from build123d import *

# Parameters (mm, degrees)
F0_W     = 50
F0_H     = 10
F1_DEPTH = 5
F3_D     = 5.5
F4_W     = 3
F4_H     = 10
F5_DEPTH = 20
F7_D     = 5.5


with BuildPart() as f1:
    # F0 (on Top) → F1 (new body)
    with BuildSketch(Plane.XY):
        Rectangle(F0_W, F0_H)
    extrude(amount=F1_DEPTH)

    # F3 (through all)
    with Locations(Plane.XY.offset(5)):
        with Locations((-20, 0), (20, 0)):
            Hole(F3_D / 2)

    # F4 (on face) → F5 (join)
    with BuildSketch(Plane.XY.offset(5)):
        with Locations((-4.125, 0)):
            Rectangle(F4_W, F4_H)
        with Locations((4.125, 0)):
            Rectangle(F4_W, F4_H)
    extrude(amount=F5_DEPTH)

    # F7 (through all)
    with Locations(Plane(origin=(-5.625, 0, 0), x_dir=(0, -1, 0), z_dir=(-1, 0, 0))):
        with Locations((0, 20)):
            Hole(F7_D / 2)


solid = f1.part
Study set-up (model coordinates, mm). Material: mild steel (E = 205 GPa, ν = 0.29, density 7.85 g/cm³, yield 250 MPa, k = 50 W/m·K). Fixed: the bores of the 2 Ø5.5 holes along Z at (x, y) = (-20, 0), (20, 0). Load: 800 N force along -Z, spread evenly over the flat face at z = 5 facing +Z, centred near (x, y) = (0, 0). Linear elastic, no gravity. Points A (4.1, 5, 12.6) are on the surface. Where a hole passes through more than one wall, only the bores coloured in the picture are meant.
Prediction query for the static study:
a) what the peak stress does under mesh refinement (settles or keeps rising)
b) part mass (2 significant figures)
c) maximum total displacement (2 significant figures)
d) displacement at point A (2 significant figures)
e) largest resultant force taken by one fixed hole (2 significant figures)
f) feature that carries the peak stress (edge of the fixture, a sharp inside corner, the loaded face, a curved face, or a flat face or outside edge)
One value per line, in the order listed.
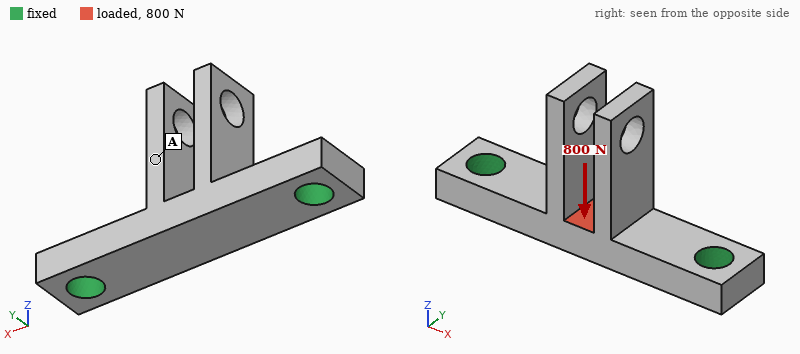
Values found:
keeps rising
26 g
17 µm
11 µm
400 N
edge of the fixture
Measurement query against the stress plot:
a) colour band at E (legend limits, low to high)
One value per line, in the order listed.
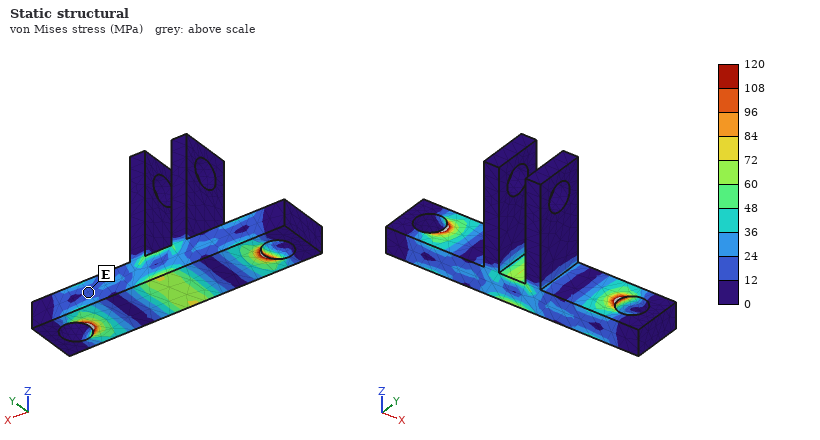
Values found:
12 to 24 MPa
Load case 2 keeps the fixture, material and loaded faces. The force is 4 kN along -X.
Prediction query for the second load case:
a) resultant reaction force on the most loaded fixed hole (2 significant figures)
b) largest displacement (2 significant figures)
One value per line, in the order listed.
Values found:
2.0 kN
9.9 µm
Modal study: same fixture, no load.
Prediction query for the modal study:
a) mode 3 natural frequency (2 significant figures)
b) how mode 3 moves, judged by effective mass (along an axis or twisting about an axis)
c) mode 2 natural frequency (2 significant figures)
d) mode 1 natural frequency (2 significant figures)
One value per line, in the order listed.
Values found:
6800 Hz
along Y
6000 Hz
5800 Hz
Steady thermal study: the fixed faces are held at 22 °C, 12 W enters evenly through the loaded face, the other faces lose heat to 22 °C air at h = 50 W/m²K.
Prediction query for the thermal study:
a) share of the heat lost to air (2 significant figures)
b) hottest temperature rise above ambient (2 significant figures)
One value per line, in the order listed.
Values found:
18 %
40 K
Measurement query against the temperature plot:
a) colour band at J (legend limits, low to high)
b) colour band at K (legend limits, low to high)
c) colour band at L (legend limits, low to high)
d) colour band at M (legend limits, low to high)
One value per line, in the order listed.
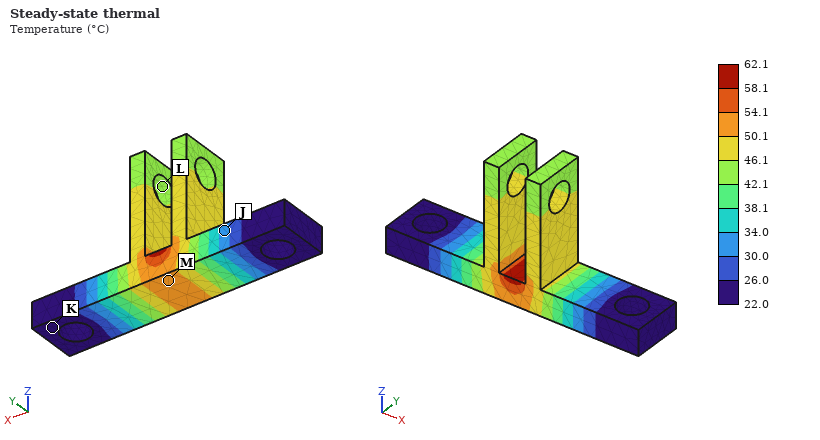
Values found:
30.0 to 34.0 °C
22.0 to 26.0 °C
42.1 to 46.1 °C
50.1 to 54.1 °C
